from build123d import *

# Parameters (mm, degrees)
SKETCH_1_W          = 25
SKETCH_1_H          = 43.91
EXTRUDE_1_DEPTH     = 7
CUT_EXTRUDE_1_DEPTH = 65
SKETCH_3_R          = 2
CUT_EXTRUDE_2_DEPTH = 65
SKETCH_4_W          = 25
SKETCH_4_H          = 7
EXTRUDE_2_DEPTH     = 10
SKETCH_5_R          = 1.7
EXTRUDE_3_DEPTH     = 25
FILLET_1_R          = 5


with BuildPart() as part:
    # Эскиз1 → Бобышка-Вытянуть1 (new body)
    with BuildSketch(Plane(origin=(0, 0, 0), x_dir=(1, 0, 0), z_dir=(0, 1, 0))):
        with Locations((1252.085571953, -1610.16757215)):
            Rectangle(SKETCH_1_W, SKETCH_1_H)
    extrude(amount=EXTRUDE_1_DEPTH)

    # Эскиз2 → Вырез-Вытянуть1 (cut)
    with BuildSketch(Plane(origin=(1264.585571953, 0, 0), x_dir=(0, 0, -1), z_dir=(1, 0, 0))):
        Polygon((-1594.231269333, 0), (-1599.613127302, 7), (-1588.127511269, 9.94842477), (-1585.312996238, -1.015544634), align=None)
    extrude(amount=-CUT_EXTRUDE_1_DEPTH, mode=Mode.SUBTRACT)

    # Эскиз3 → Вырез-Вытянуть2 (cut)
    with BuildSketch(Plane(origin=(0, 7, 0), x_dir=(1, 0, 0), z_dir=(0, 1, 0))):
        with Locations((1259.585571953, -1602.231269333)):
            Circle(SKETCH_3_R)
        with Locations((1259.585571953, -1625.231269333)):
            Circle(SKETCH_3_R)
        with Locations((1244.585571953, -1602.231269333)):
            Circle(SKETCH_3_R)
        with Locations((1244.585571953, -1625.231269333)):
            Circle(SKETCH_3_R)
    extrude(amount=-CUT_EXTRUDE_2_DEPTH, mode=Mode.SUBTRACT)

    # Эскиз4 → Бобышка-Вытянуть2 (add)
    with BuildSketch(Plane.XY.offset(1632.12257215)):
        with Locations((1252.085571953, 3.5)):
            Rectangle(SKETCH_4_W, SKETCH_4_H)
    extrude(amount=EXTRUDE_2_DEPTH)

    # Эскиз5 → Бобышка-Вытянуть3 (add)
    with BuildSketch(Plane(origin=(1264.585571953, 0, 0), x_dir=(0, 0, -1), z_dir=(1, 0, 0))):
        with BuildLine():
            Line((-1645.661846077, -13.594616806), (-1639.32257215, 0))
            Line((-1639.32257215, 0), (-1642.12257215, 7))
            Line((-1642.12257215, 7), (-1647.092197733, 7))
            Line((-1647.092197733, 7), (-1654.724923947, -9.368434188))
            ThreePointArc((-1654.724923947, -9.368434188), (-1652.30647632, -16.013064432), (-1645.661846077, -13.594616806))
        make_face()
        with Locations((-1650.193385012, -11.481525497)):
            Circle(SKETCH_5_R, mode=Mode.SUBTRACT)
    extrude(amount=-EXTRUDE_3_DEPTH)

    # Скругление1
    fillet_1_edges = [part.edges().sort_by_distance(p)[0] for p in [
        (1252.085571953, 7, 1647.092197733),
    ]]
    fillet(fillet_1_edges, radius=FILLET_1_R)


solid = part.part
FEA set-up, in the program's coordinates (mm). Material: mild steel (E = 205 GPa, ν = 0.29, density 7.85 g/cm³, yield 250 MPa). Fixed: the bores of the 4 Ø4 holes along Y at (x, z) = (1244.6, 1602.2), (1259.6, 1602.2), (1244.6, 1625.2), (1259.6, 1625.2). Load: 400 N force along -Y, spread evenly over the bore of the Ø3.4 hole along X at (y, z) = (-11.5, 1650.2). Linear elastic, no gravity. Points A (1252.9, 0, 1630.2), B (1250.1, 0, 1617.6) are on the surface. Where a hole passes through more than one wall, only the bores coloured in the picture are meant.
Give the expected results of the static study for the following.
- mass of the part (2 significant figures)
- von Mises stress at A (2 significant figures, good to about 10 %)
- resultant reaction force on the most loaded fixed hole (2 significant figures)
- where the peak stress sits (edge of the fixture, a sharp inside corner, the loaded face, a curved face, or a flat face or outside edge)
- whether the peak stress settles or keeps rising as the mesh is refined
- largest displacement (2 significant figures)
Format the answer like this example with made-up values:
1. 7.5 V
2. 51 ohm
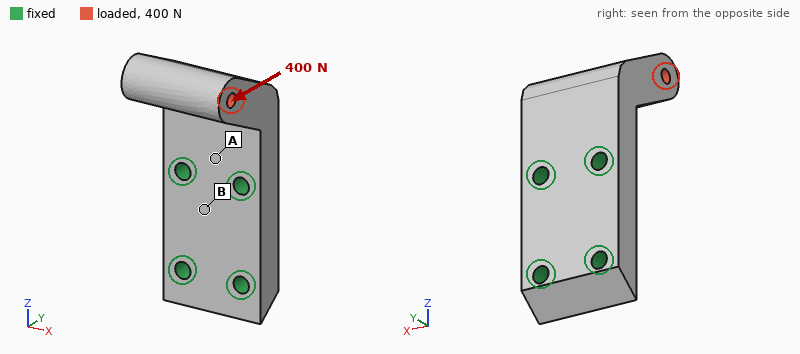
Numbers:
1. 99 g
2. 30 MPa
3. 230 N
4. edge of the fixture
5. keeps rising
6. 22 µm
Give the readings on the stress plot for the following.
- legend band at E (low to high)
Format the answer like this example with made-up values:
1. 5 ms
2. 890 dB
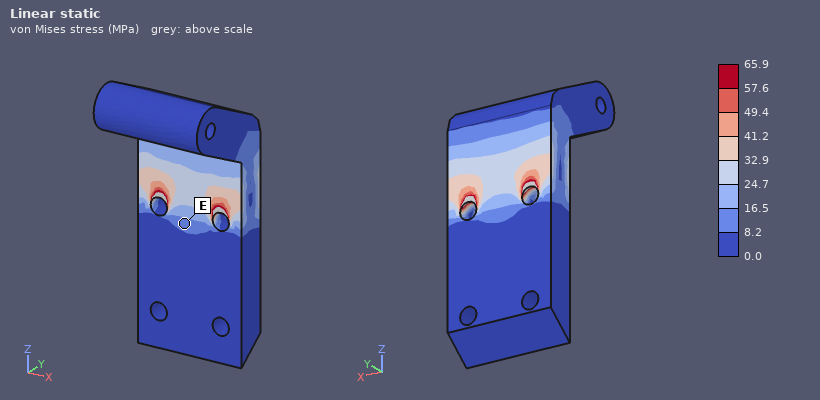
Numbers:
1. 8.2 to 16.5 MPa
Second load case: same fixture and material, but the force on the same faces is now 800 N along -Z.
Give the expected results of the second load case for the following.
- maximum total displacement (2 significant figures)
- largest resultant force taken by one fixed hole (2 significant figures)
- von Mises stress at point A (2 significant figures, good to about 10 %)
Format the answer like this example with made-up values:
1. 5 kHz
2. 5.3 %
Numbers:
1. 40 µm
2. 380 N
3. 49 MPa
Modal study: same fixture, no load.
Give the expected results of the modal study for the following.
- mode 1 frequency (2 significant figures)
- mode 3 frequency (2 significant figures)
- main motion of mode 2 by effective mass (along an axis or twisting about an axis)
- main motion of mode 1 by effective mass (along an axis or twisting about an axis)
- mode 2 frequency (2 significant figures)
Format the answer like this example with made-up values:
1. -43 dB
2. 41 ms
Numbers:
1. 4100 Hz
2. 16 kHz
3. along X
4. along Y
5. 7900 Hz
